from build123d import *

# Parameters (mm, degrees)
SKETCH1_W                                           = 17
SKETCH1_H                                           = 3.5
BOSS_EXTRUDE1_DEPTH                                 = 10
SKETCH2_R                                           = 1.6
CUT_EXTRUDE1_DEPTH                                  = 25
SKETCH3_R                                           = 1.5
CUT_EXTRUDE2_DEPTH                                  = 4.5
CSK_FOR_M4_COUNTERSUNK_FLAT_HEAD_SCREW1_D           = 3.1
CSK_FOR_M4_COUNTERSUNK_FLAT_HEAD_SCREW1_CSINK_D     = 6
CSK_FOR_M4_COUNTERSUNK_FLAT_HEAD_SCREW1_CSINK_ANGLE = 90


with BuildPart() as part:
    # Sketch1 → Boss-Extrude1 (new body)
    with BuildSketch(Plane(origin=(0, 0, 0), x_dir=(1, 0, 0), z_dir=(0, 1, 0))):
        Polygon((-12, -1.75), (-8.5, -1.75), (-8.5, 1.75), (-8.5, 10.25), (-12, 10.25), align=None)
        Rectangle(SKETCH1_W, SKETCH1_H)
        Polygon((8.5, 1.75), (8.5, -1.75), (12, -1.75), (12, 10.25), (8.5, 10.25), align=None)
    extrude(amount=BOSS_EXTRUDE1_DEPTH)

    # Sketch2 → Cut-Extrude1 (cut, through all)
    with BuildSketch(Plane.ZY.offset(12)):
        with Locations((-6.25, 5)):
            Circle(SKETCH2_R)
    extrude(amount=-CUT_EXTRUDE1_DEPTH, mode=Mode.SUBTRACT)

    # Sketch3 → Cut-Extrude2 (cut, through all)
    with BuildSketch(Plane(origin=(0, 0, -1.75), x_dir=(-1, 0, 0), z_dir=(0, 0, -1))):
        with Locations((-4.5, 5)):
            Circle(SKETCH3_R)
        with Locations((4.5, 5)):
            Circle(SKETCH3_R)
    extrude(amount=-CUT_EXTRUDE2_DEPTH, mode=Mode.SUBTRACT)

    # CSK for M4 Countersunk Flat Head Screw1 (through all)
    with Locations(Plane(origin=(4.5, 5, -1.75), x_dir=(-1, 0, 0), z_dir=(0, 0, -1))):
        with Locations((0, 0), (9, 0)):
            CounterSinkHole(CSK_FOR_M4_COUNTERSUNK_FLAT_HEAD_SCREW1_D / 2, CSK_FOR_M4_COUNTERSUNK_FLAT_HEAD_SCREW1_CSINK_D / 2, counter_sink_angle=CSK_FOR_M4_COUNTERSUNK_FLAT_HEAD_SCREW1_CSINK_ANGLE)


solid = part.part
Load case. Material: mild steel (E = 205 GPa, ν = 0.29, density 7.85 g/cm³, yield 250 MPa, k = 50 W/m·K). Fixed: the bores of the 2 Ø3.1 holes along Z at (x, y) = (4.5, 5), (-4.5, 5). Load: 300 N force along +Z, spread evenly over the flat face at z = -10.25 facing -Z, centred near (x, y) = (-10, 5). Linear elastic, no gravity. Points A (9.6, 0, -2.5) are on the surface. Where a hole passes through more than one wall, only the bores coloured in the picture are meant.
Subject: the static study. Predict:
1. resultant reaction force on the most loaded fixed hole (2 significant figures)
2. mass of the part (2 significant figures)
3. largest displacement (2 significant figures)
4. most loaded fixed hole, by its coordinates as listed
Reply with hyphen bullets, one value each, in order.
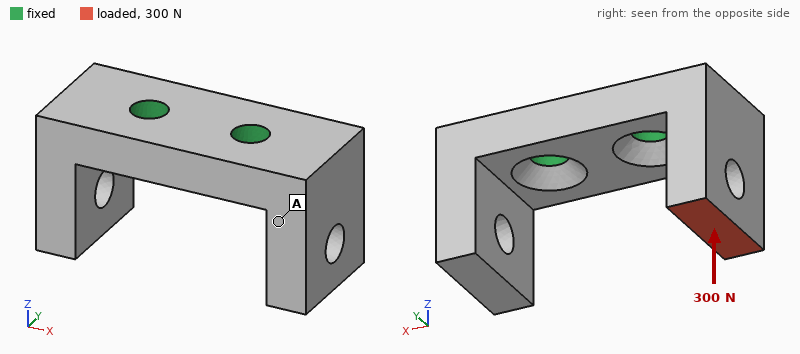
- 370 N
- 10 g
- 12 µm
- (-4.5, 5)
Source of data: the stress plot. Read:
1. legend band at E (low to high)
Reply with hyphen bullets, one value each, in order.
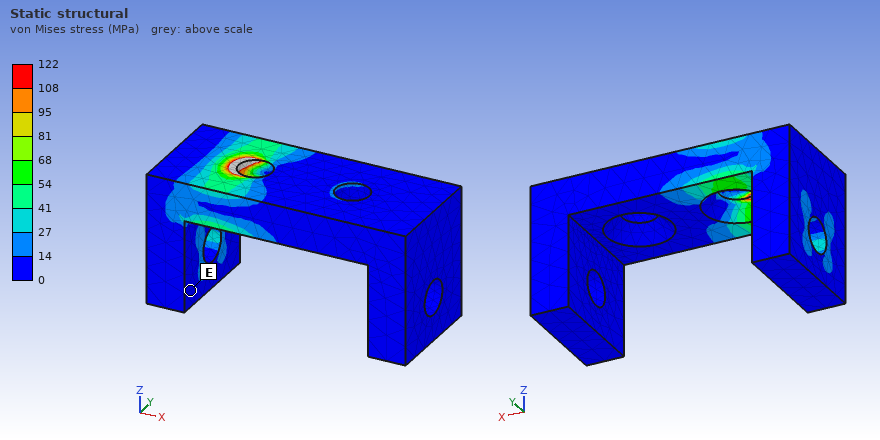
- 0 to 14 MPa
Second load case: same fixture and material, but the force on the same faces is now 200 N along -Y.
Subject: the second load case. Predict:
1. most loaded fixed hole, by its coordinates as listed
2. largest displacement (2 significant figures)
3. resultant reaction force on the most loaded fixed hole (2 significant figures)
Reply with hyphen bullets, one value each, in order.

- (-4.5, 5)
- 19 µm
- 240 N
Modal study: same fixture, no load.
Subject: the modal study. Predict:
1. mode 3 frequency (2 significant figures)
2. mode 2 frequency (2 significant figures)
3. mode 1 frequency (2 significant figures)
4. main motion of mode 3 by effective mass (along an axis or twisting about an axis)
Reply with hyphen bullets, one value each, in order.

- 16 kHz
- 13 kHz
- 13 kHz
- along Y
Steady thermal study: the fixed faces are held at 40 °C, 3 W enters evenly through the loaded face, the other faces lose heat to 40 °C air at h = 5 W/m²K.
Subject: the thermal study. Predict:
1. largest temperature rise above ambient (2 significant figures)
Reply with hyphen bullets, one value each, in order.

- 29 K
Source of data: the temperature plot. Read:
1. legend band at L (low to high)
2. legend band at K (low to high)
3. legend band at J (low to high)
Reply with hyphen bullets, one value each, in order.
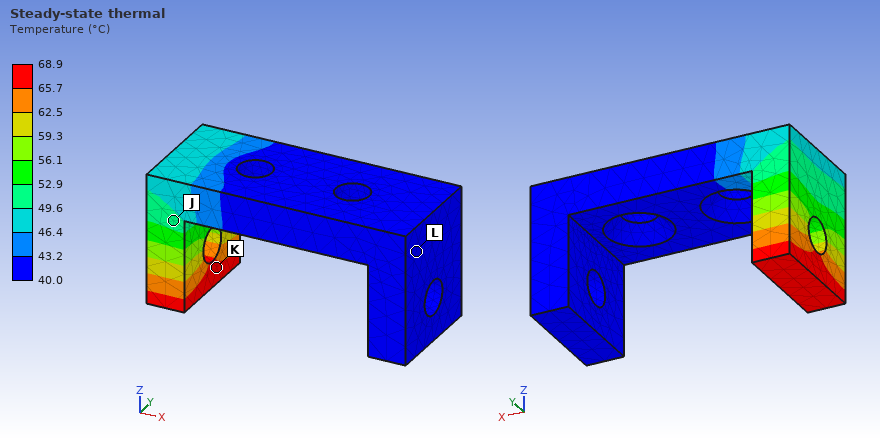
- 40.0 to 43.2 °C
- 65.7 to 68.9 °C
- 49.6 to 52.9 °C
